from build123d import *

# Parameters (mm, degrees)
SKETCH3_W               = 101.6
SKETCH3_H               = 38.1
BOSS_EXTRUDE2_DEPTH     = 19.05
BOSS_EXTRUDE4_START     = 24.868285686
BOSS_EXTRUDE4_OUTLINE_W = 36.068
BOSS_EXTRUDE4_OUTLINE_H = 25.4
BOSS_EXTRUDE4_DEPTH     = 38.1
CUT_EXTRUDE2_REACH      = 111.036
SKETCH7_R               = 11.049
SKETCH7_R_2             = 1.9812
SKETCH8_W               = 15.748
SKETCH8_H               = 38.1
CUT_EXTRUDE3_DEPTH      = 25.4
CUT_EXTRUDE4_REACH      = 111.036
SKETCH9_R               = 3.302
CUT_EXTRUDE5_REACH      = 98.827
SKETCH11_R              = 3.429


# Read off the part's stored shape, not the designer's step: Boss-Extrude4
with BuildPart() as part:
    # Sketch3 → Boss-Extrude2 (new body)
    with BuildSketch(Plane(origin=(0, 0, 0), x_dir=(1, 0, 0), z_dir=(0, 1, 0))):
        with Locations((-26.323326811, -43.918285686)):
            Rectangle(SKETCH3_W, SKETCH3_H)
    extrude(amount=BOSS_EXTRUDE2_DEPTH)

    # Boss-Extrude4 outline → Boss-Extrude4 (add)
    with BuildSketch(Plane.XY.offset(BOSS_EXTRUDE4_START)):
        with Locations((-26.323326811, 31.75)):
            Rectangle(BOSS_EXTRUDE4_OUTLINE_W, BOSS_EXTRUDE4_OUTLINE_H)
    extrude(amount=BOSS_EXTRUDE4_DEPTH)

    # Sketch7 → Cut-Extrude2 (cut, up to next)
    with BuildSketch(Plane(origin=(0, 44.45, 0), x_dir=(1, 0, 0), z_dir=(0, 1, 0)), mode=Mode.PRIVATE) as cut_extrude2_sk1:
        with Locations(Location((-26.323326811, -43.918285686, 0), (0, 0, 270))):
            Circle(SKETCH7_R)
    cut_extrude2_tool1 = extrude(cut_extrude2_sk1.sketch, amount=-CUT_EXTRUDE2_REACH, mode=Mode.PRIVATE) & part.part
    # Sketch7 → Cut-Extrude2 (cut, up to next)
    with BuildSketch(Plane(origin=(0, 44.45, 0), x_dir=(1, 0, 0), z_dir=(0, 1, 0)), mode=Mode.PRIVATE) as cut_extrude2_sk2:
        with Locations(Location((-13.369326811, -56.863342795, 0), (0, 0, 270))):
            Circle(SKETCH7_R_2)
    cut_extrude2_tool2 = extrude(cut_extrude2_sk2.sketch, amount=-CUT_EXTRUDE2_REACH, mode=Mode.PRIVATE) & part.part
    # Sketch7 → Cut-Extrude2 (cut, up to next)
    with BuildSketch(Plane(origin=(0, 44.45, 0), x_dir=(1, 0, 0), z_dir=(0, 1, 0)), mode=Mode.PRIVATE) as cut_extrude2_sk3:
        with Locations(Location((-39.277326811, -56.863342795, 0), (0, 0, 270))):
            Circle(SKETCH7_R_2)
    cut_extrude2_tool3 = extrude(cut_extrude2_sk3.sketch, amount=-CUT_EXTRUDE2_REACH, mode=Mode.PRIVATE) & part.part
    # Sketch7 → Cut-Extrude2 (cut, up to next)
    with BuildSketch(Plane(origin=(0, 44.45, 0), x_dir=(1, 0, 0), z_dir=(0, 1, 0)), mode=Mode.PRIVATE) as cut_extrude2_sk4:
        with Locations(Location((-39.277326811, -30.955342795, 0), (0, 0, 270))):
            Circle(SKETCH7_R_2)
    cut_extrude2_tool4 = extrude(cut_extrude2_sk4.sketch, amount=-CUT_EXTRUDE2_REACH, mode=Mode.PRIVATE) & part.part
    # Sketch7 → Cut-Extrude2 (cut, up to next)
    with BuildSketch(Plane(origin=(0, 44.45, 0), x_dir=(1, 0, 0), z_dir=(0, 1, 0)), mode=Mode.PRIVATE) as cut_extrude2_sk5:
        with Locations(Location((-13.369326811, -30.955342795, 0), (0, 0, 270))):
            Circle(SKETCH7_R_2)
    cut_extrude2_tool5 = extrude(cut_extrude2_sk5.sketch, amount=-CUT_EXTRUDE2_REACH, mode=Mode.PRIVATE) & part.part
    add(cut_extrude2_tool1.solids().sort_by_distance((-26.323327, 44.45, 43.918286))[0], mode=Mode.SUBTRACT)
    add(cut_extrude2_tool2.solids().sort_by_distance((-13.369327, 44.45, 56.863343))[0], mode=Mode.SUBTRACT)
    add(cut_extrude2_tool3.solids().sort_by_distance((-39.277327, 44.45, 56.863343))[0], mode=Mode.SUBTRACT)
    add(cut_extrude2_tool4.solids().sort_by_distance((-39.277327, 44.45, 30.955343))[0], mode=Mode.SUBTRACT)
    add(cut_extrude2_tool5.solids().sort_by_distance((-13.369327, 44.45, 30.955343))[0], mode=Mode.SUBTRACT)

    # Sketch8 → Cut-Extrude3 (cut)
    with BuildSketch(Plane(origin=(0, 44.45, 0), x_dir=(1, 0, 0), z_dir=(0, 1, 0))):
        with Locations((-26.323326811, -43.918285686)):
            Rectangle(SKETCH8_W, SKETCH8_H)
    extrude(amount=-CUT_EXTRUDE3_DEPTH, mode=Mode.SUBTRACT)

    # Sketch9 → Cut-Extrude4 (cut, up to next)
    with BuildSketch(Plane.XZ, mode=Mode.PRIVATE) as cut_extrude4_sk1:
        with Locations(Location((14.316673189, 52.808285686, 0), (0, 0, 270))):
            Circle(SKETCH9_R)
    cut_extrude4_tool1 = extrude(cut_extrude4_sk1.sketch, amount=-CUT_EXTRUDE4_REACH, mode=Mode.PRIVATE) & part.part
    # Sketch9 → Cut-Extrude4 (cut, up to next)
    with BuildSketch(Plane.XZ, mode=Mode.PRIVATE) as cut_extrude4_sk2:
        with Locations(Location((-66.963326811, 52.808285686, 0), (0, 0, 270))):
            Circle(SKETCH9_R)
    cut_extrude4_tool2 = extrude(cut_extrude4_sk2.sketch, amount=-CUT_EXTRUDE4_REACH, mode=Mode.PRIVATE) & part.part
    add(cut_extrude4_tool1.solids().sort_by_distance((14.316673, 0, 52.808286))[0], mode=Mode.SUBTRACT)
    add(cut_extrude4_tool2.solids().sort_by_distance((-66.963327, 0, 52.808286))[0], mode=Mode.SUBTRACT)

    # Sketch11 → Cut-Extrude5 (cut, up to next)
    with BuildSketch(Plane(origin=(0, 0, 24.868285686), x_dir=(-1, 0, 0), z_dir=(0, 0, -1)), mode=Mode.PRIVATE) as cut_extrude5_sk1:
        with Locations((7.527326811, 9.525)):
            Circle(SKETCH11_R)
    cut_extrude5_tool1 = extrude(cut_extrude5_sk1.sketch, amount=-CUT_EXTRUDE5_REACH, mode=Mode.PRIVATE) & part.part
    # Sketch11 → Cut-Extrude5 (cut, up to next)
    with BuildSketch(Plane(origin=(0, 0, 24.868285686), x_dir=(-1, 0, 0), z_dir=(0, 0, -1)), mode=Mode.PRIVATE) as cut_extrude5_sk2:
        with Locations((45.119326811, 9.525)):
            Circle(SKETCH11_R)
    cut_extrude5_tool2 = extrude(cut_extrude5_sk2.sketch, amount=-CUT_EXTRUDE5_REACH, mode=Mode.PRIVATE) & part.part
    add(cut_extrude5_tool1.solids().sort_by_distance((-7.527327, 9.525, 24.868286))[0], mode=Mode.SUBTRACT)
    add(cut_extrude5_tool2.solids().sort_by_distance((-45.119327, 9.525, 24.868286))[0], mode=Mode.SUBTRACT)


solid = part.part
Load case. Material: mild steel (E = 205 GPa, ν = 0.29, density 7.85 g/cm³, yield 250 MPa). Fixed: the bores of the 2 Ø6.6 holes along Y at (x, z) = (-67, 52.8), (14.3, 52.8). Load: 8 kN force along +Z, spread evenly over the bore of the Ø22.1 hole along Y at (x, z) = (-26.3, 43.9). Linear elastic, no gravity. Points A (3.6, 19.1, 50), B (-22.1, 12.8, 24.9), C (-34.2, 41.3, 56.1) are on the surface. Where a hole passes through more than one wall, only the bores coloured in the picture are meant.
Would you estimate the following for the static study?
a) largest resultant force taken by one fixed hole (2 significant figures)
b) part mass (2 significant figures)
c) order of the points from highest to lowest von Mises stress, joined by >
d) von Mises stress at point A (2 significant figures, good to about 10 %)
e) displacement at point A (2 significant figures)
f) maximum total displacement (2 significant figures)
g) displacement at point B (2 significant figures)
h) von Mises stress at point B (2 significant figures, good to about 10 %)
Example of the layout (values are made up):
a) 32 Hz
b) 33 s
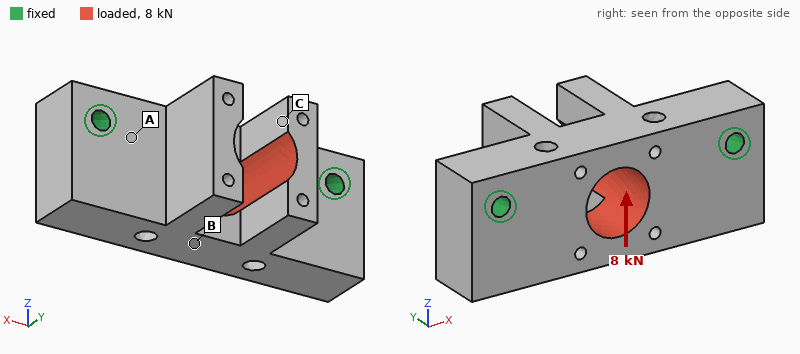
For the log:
a) 4.5 kN
b) 610 g
c) A > B > C
d) 32 MPa
e) 3.4 µm
f) 19 µm
g) 9.4 µm
h) 24 MPa
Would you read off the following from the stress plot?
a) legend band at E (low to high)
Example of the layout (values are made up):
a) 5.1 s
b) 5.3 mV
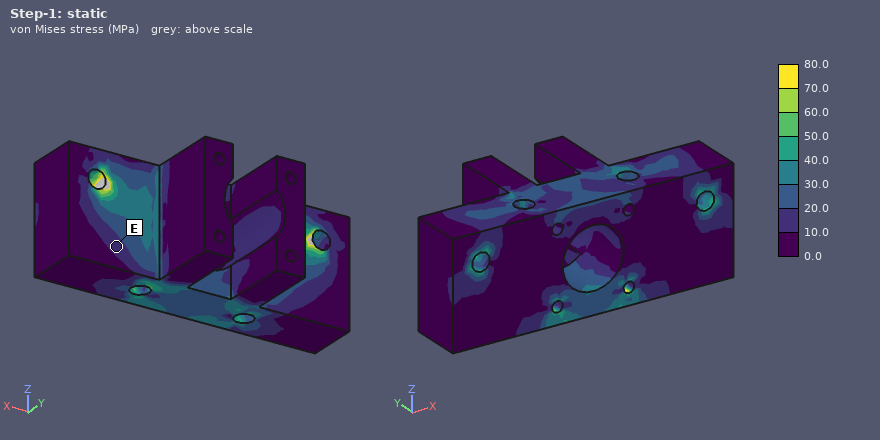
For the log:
a) 10.0 to 20.0 MPa
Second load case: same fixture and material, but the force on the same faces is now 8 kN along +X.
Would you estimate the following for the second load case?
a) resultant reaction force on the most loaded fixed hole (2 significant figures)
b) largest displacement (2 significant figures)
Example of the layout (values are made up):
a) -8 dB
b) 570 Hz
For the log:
a) 4.2 kN
b) 15 µm
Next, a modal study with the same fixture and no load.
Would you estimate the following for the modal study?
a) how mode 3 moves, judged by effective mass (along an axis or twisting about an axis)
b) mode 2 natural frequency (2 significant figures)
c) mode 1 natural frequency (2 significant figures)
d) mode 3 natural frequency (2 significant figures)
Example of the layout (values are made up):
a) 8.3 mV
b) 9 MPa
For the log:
a) along X
b) 6800 Hz
c) 5900 Hz
d) 8200 Hz
